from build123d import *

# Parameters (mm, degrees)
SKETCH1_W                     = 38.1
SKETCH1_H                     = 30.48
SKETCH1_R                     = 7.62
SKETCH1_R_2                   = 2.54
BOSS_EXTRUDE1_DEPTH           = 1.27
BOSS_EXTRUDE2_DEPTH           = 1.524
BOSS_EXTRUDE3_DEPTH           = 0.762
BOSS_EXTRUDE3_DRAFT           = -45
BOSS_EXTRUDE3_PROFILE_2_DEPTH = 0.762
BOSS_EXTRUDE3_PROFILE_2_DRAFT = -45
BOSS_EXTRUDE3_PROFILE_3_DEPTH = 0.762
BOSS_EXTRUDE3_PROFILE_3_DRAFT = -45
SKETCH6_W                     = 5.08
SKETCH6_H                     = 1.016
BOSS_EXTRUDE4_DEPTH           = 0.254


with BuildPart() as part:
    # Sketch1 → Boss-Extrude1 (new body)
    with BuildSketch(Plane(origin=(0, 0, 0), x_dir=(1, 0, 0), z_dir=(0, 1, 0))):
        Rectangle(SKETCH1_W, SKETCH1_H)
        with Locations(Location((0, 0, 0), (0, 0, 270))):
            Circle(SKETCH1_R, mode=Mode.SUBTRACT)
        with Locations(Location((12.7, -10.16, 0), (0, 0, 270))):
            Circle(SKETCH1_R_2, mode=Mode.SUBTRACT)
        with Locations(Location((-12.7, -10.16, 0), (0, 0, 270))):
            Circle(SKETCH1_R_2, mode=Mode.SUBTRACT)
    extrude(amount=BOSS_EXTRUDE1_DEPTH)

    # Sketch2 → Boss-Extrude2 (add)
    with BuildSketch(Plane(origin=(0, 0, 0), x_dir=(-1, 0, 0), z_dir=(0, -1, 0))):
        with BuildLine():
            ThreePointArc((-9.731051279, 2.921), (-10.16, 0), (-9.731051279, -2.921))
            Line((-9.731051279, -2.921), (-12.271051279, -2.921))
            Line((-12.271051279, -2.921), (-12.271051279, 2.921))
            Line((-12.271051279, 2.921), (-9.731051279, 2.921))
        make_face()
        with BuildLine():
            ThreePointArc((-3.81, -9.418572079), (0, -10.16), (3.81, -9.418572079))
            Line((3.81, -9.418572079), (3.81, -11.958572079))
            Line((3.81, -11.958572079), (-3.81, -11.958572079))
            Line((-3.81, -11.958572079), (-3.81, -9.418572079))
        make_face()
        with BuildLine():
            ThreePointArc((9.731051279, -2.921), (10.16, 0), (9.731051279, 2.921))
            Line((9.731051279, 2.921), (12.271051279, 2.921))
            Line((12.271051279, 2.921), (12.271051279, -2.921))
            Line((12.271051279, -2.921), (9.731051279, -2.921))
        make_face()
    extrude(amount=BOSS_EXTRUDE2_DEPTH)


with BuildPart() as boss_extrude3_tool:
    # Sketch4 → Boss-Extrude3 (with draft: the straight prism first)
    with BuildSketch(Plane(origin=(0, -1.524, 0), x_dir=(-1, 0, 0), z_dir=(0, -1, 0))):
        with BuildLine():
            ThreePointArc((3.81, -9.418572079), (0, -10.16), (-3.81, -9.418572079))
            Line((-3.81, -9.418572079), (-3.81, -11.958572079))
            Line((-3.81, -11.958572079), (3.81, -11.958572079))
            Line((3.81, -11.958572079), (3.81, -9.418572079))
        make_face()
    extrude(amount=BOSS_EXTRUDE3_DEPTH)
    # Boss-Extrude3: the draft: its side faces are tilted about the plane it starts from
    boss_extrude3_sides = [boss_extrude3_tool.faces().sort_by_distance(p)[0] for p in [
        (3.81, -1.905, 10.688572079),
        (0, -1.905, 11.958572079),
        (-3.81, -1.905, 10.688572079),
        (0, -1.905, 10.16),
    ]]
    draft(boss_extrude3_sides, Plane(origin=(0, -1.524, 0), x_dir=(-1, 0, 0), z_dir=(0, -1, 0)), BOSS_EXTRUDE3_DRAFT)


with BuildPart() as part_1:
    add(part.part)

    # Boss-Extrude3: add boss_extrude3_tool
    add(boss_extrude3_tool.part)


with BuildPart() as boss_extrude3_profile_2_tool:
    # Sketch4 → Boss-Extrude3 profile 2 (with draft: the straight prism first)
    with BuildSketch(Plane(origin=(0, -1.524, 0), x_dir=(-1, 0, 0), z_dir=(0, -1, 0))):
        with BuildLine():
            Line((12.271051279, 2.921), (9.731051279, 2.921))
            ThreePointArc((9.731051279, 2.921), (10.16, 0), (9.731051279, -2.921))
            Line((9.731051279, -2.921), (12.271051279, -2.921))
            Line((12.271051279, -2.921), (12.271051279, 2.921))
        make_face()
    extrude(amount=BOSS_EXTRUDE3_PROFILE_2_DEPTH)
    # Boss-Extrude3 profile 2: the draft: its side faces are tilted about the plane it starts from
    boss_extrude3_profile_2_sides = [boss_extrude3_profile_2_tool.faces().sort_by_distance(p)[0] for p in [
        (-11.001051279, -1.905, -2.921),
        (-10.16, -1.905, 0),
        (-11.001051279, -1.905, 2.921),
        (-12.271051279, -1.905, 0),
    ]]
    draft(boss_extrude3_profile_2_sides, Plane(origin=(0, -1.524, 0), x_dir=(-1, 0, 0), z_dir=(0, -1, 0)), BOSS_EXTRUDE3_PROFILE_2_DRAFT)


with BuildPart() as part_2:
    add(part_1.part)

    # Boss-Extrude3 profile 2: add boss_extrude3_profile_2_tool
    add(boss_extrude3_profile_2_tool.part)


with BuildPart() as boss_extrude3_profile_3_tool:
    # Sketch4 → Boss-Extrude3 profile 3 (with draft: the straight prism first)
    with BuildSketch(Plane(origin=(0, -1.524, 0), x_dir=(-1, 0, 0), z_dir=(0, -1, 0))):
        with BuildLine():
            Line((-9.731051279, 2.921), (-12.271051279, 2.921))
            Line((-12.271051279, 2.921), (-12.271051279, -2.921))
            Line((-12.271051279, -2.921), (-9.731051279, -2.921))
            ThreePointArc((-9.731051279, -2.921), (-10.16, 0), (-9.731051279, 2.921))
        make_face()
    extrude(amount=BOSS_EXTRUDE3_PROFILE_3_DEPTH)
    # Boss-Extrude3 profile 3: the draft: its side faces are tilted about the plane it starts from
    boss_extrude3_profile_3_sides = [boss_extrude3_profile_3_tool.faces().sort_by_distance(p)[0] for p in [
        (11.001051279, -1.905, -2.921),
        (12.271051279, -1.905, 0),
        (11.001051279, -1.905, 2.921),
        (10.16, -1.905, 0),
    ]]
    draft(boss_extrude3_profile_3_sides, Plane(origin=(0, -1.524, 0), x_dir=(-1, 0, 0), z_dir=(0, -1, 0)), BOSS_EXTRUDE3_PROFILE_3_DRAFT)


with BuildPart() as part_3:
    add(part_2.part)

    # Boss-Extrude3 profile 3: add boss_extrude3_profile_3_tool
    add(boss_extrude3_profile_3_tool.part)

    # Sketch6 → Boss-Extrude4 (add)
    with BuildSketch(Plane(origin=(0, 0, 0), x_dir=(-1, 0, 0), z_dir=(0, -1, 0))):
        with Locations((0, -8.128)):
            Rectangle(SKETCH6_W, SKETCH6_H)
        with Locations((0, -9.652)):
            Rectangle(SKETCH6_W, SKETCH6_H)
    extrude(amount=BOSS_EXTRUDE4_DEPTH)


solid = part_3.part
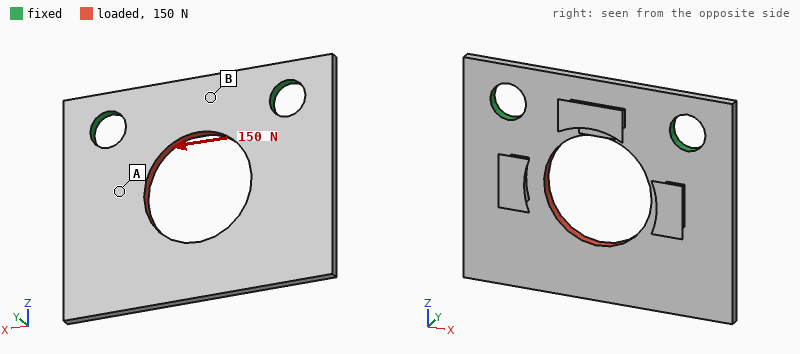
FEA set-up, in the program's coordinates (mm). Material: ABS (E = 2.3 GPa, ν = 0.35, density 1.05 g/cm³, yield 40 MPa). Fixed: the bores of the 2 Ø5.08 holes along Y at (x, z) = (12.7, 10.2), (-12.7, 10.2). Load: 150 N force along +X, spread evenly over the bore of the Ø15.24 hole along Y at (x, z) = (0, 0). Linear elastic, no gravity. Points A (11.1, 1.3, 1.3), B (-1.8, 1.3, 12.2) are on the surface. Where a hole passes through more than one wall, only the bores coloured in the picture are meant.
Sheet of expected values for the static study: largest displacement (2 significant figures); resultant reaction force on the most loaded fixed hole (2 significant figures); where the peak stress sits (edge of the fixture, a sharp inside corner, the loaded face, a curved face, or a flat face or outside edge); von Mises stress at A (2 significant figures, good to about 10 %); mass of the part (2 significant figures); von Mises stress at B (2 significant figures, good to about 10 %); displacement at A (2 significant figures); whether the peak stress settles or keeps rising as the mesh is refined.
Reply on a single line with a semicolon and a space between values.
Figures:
0.15 mm; 84 N; edge of the fixture; 7.0 MPa; 1.4 g; 4.1 MPa; 0.058 mm; keeps rising
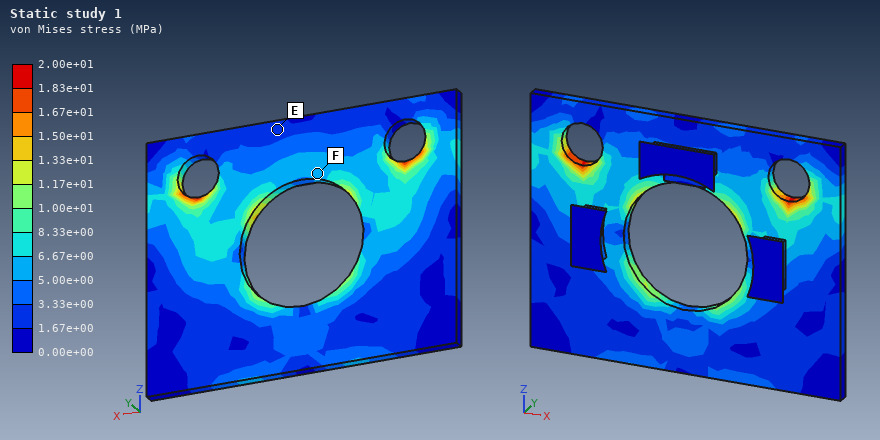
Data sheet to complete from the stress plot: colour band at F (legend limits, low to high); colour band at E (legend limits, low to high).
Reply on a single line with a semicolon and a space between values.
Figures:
5.00e+00 to 6.67e+00 MPa; 1.67e+00 to 3.33e+00 MPa
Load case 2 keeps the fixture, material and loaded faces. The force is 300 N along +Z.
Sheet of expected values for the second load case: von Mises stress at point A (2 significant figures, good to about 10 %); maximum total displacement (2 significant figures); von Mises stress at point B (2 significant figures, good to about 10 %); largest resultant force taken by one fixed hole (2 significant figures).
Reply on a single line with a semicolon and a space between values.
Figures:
11 MPa; 0.13 mm; 3.8 MPa; 150 N
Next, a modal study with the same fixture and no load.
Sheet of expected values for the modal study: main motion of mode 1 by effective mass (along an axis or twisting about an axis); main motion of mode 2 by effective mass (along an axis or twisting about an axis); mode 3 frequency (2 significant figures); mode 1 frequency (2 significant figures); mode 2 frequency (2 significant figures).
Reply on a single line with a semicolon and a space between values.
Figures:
along Y; twisting about Z; 1900 Hz; 500 Hz; 900 Hz
